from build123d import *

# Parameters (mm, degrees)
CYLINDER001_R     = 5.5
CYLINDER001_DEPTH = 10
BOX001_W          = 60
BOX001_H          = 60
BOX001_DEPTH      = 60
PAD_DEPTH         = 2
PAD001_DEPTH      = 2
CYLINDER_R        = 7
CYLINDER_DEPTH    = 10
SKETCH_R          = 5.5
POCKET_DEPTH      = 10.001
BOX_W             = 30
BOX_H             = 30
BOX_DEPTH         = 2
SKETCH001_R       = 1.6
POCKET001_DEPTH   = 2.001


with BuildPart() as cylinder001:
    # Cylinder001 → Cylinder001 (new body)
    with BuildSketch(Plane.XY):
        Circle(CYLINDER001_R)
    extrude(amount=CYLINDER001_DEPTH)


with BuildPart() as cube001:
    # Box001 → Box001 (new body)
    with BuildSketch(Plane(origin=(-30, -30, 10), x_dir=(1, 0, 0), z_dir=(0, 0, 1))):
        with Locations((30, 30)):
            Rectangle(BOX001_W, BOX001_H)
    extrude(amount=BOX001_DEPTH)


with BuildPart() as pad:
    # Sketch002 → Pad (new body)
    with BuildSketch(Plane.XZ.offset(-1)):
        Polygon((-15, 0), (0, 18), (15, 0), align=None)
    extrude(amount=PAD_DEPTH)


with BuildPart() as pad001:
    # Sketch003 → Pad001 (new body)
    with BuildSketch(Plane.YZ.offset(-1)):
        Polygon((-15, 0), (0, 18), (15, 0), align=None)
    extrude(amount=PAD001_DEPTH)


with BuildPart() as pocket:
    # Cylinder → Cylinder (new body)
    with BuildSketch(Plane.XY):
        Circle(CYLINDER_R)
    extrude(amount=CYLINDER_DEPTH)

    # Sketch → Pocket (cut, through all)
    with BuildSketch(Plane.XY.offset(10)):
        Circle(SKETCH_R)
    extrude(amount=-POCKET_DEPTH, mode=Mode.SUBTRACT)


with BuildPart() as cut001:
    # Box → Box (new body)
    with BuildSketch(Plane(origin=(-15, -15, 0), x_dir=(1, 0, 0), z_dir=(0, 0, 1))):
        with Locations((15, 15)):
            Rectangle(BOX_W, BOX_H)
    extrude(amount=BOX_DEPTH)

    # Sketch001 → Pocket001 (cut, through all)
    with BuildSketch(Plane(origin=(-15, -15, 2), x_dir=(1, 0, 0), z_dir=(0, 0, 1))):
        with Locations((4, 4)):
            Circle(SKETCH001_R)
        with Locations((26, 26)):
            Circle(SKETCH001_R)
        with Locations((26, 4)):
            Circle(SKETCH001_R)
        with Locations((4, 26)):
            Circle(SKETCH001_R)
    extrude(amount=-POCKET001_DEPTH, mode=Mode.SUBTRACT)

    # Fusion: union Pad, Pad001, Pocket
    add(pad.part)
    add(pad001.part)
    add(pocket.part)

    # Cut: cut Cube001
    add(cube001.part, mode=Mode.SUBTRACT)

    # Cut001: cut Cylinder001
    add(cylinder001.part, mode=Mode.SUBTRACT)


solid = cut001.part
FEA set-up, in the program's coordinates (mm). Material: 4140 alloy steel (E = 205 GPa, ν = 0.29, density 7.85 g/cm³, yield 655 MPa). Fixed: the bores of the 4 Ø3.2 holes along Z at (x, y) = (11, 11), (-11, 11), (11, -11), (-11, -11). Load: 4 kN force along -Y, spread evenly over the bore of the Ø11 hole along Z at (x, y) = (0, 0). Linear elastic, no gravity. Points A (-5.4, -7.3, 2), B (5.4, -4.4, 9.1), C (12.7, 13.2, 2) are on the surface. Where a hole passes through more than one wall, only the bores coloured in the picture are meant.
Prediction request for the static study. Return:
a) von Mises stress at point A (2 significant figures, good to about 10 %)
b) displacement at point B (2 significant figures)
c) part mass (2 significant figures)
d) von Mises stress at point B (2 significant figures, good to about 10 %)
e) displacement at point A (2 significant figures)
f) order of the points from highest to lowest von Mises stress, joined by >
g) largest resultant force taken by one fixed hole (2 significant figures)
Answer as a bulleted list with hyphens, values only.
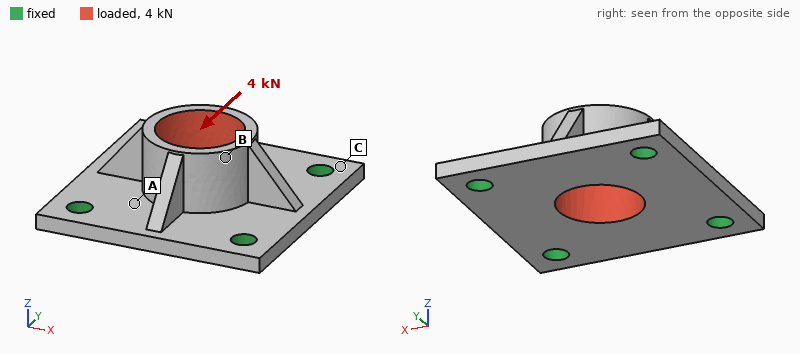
- 130 MPa
- 23 µm
- 17 g
- 60 MPa
- 8.6 µm
- A > B > C
- 1.1 kN
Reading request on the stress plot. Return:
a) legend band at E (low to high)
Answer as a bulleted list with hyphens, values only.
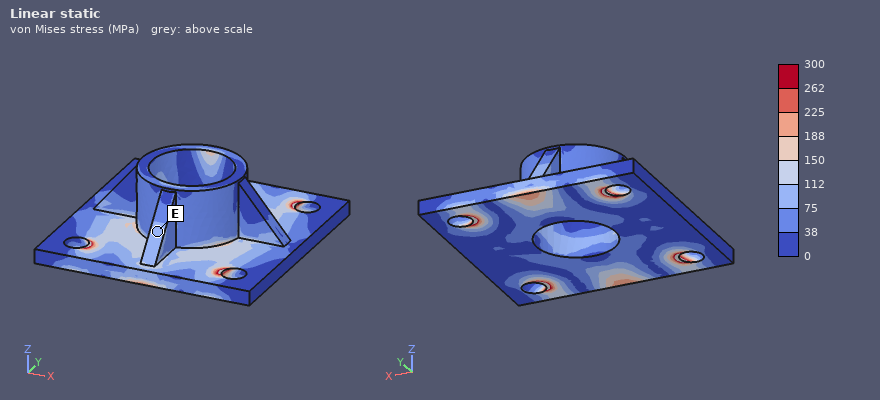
- 75 to 112 MPa
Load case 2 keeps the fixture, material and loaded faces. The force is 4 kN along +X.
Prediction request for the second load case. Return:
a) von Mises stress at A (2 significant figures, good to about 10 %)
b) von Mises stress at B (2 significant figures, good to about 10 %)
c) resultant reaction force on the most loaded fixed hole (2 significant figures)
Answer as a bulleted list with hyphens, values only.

- 140 MPa
- 60 MPa
- 1.1 kN
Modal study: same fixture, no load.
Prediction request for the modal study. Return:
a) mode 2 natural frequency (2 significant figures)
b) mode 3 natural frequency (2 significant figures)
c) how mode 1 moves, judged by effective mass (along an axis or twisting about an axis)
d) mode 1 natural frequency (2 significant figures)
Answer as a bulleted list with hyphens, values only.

- 20 kHz
- 20 kHz
- along Z
- 17 kHz
